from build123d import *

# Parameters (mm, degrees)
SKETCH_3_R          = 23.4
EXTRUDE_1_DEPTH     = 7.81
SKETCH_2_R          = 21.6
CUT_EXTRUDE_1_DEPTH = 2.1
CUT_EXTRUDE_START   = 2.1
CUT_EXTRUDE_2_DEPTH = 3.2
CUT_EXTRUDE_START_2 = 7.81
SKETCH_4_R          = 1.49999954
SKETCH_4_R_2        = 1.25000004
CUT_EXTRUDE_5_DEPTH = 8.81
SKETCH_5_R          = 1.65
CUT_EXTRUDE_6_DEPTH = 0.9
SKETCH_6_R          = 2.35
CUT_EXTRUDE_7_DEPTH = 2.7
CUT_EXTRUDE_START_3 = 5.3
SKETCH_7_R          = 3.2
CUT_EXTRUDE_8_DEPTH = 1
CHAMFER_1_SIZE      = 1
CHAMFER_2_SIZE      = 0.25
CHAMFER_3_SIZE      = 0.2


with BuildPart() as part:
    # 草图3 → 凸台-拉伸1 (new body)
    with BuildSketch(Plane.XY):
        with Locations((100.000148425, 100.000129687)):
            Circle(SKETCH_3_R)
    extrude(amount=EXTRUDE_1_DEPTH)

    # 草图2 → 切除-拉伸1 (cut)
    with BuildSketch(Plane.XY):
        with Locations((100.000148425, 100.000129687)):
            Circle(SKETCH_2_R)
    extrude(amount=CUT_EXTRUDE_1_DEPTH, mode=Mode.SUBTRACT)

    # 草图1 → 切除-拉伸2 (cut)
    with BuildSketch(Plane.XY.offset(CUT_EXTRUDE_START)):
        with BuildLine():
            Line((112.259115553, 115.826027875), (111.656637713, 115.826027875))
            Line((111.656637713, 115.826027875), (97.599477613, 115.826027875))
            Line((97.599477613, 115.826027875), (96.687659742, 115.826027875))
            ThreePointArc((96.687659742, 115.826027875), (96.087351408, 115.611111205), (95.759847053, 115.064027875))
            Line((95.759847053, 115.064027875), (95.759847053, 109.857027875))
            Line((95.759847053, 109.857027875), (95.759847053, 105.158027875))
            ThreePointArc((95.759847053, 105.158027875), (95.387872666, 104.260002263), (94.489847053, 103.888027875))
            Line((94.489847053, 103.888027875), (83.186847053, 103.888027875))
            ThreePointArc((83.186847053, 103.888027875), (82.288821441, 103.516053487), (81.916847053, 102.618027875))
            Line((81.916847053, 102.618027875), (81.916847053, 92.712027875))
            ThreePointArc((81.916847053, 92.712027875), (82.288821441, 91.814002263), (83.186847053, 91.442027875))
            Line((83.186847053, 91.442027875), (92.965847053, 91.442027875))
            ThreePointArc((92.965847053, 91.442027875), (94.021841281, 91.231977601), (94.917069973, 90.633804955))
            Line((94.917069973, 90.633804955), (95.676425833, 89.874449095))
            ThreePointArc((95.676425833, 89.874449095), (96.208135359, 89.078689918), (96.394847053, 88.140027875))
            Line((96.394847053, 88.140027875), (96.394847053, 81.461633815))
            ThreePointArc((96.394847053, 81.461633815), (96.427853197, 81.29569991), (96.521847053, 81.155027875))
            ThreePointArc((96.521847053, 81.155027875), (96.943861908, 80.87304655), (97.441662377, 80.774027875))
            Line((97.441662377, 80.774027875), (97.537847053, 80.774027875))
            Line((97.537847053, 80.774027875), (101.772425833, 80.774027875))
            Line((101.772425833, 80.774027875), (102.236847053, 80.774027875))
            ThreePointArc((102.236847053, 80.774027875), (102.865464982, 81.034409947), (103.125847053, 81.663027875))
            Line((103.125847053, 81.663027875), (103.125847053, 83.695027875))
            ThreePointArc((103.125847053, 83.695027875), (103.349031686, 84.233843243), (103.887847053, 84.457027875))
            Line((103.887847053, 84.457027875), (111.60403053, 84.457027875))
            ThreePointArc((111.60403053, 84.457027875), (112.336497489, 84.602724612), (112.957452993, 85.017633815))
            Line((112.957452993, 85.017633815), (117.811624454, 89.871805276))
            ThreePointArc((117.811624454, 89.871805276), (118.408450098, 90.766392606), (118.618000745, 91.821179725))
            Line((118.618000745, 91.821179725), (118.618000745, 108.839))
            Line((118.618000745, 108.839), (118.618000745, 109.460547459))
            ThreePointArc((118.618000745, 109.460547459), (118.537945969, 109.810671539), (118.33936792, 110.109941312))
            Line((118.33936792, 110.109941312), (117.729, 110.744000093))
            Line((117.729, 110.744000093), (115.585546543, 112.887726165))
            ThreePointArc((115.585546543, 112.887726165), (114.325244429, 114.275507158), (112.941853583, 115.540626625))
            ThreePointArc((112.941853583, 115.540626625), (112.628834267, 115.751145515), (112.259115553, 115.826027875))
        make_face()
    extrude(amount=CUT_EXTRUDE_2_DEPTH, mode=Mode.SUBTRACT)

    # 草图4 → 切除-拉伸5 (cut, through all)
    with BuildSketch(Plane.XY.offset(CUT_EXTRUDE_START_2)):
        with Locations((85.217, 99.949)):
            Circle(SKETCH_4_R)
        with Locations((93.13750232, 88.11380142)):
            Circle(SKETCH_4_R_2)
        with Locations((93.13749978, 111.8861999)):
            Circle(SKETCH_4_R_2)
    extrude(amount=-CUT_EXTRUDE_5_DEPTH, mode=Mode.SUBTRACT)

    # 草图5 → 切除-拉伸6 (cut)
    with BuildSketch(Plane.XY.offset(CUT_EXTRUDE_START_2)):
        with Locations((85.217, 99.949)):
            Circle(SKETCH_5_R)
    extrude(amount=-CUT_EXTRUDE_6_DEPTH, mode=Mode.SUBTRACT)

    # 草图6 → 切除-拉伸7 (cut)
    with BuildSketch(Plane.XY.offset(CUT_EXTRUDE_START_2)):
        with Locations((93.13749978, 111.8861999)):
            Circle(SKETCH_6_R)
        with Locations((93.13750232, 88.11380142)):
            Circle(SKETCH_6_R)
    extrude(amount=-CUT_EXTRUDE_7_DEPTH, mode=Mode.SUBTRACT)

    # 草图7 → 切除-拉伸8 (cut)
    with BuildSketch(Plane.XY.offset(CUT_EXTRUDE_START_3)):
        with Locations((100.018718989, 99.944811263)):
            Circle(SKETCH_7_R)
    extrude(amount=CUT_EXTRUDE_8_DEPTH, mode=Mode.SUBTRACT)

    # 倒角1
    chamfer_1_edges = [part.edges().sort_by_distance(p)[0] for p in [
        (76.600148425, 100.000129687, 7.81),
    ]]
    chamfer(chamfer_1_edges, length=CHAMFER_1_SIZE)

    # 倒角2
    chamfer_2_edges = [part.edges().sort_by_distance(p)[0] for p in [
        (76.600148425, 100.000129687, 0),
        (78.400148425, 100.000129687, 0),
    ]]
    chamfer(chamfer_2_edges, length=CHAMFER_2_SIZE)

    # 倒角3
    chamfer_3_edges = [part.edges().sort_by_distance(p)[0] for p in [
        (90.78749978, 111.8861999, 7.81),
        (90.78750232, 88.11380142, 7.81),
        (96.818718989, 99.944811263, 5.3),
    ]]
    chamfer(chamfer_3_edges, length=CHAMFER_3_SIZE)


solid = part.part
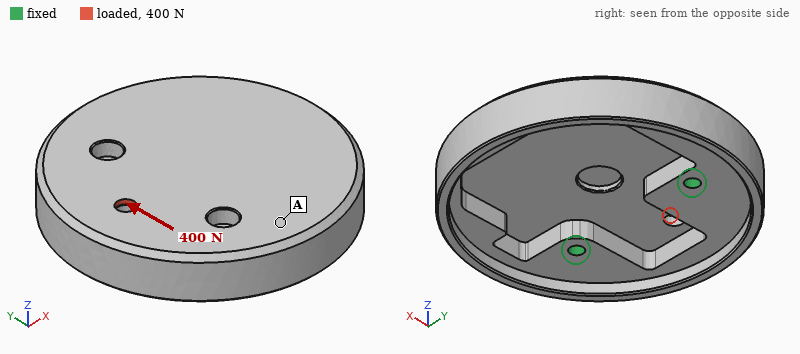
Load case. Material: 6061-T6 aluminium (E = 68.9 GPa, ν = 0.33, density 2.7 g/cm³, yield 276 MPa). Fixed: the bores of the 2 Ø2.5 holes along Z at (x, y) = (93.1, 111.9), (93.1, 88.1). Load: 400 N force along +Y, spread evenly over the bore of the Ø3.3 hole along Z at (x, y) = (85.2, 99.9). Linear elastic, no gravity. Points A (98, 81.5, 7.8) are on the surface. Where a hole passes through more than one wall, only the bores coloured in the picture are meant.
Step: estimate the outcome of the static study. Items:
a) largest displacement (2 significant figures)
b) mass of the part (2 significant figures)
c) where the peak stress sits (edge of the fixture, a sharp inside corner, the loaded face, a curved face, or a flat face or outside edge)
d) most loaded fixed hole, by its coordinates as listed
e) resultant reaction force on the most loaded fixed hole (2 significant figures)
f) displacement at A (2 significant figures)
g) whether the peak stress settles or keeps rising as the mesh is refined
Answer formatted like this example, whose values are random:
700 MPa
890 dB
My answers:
3.7 µm
20 g
a sharp inside corner
(93.1, 111.9)
260 N
1.3 µm
keeps rising
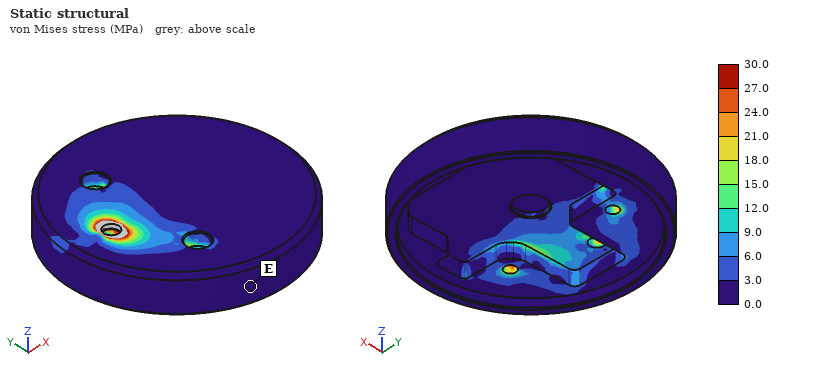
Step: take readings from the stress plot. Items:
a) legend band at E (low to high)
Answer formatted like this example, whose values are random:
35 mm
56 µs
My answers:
0.0 to 3.0 MPa
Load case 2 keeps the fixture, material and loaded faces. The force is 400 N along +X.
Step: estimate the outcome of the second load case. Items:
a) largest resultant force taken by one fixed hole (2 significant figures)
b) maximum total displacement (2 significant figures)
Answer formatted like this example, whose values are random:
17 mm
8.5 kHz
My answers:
210 N
21 µm
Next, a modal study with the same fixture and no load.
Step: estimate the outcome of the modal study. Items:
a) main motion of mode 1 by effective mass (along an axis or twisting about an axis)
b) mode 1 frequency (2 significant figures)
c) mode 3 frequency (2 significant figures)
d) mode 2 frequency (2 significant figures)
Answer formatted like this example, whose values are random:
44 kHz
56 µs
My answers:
along Z
2900 Hz
10 kHz
7000 Hz
